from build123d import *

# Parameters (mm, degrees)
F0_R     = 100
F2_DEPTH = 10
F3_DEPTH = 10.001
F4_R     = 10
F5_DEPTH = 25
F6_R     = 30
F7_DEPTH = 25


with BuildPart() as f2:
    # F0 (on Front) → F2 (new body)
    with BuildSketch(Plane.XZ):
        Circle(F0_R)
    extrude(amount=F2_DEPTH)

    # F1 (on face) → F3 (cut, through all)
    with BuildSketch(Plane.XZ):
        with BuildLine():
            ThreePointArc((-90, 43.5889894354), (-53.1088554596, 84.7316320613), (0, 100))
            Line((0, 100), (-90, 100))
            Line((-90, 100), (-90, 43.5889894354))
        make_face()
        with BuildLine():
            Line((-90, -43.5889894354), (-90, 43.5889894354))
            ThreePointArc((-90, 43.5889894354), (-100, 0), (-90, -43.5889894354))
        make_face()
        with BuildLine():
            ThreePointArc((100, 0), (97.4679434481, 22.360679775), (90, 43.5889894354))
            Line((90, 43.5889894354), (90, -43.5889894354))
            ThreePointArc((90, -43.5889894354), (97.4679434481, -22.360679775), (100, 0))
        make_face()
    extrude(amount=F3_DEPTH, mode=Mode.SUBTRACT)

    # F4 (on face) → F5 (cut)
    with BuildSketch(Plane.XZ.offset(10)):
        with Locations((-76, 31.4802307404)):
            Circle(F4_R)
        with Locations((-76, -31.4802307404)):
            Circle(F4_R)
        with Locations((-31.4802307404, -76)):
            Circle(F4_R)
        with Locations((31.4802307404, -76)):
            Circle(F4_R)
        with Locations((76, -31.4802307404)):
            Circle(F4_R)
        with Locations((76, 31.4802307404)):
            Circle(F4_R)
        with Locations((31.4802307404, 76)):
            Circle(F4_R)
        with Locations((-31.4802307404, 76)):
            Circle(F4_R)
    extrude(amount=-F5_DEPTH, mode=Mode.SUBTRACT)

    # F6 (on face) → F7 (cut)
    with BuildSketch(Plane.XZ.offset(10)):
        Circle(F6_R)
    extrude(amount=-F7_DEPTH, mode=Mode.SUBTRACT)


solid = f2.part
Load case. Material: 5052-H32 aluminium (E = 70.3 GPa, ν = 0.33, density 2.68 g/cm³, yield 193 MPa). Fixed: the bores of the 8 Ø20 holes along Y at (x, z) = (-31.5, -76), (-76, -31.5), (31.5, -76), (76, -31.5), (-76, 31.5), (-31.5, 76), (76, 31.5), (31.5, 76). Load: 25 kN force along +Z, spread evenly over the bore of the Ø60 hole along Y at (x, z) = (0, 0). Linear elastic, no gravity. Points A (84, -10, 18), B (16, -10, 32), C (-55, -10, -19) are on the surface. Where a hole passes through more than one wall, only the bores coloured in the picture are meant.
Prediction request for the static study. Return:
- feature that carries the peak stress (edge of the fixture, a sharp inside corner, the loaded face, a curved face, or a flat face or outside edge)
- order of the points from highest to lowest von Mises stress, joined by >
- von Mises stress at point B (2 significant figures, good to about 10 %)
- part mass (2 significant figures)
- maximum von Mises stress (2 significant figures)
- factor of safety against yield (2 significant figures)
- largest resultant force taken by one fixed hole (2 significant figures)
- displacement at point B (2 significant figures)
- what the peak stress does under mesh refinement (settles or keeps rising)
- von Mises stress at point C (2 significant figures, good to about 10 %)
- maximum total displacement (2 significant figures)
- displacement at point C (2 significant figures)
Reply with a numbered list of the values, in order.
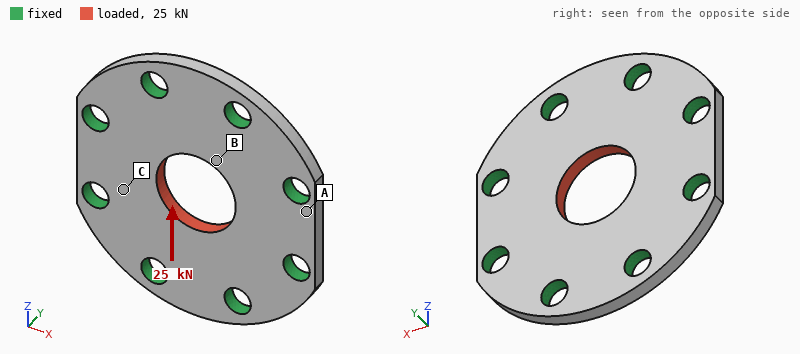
1. the loaded face
2. B > C > A
3. 13 MPa
4. 670 g
5. 23 MPa
6. 8.4
7. 4.8 kN
8. 7.3 µm
9. settles
10. 6.8 MPa
11. 9.1 µm
12. 2.0 µm
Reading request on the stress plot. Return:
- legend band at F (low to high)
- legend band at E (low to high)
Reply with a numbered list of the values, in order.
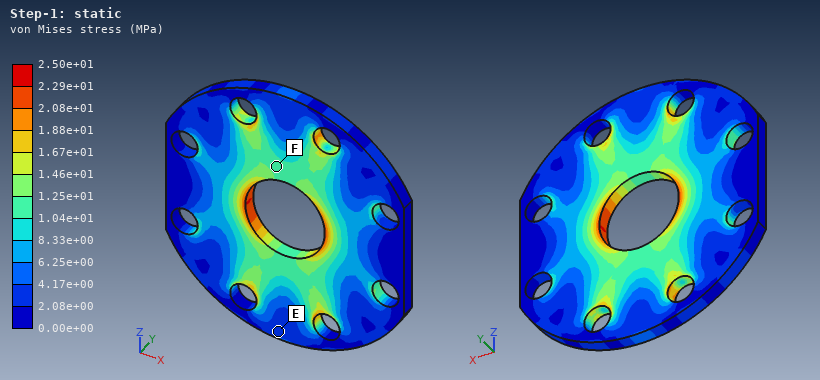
1. 1.04e+01 to 1.25e+01 MPa
2. 2.08e+00 to 4.17e+00 MPa
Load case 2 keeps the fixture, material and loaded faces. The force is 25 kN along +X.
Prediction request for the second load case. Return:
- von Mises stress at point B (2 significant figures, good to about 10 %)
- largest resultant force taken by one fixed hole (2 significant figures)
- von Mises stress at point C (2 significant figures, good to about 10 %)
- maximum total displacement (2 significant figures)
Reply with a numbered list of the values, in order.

1. 14 MPa
2. 4.9 kN
3. 13 MPa
4. 9.2 µm
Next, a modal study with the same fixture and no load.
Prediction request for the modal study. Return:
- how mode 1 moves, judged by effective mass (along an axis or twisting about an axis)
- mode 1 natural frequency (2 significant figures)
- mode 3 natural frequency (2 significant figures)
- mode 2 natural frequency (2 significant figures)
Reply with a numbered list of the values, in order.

1. along Y
2. 5100 Hz
3. 7100 Hz
4. 7100 Hz
